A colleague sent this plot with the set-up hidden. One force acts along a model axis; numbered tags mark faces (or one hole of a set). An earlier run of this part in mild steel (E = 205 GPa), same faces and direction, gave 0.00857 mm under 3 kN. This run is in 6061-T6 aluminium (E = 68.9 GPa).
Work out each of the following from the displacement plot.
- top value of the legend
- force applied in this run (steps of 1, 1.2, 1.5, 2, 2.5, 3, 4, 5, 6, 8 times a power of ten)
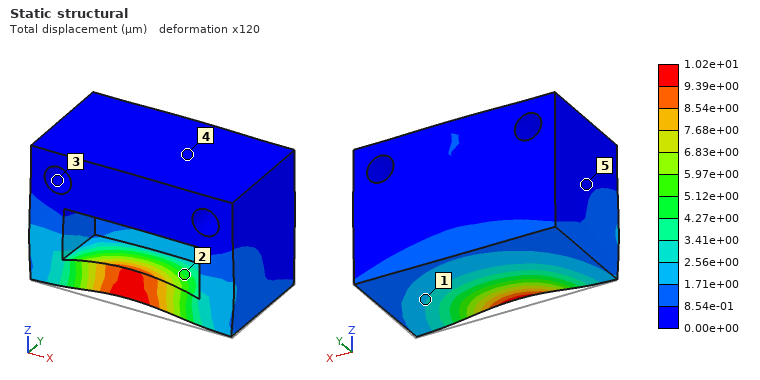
1.02e+01 µm
1.2 kN
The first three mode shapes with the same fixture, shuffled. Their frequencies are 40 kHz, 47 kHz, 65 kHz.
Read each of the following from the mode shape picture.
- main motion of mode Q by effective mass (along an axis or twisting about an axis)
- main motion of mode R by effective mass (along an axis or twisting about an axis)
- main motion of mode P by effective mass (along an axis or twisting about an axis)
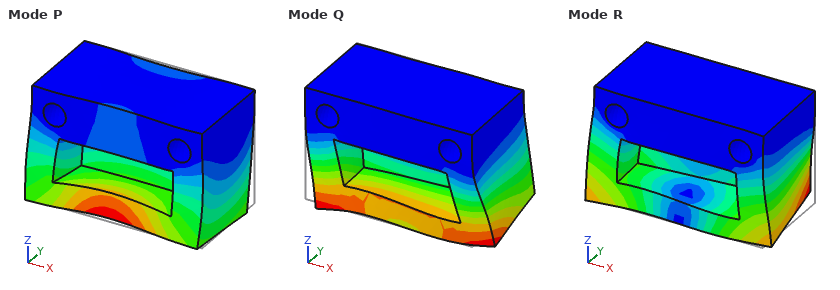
along X
along X
along Y
